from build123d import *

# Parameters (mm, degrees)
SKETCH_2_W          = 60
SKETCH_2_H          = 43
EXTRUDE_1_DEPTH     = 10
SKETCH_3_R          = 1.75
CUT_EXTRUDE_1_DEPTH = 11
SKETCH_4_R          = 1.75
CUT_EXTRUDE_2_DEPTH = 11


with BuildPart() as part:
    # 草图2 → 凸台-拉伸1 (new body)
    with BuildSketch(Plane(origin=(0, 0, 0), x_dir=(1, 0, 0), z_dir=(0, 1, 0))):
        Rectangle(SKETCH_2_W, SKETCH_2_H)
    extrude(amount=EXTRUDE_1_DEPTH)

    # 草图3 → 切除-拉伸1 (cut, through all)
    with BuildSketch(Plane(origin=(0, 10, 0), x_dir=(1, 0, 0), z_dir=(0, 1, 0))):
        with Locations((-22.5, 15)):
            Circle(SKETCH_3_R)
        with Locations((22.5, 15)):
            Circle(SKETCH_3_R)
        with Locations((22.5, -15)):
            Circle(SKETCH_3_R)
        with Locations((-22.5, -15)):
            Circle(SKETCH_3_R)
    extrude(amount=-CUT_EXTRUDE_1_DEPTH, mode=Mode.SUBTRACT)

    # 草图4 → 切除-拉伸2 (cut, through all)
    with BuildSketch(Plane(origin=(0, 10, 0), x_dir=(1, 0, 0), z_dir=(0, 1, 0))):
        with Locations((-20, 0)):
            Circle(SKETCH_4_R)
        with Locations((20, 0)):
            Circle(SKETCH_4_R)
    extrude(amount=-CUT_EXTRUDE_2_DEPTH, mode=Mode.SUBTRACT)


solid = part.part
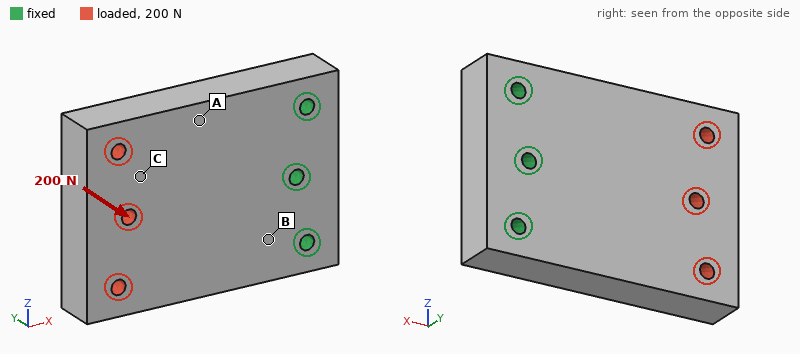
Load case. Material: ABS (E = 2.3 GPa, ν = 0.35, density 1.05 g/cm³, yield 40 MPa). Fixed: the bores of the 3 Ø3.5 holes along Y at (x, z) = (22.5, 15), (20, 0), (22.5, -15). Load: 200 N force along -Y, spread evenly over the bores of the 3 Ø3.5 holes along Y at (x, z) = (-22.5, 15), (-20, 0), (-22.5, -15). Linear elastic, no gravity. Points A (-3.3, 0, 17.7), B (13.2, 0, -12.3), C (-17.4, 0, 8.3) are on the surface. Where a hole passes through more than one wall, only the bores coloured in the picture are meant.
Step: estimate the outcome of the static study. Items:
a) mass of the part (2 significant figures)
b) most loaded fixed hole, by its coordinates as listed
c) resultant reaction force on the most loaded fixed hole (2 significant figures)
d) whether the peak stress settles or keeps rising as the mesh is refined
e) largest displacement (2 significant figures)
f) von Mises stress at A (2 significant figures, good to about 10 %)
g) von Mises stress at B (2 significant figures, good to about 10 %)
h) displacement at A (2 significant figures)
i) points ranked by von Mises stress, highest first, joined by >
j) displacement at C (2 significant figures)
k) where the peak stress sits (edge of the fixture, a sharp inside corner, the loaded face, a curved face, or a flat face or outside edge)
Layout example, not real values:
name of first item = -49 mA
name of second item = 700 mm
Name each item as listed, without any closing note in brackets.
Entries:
mass of the part = 26 g
most loaded fixed hole, by its coordinates as listed = (20, 0)
resultant reaction force on the most loaded fixed hole = 210 N
whether the peak stress settles or keeps rising as the mesh is refined = keeps rising
largest displacement = 0.87 mm
von Mises stress at A = 5.1 MPa
von Mises stress at B = 8.8 MPa
displacement at A = 0.29 mm
points ranked by von Mises stress, highest first, joined by > = B > A > C
displacement at C = 0.59 mm
where the peak stress sits = edge of the fixture
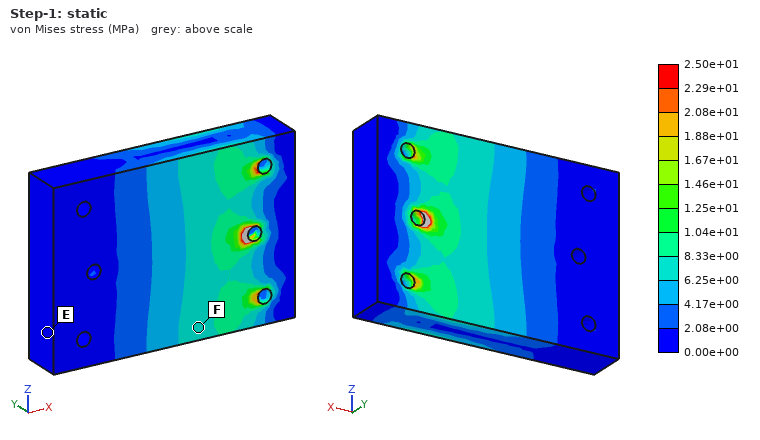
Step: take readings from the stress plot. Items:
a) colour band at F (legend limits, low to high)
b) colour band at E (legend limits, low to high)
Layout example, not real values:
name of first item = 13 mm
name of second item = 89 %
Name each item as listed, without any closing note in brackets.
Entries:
colour band at F = 6.25e+00 to 8.33e+00 MPa
colour band at E = 0.00e+00 to 2.08e+00 MPa
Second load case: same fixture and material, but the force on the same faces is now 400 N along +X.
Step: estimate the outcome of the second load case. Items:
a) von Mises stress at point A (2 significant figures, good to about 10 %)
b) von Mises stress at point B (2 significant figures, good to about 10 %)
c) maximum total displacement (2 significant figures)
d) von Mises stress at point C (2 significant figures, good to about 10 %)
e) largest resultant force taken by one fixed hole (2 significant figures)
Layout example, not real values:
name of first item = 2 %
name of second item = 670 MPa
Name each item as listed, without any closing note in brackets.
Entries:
von Mises stress at point A = 0.88 MPa
von Mises stress at point B = 0.94 MPa
maximum total displacement = 21 µm
von Mises stress at point C = 0.68 MPa
largest resultant force taken by one fixed hole = 140 N
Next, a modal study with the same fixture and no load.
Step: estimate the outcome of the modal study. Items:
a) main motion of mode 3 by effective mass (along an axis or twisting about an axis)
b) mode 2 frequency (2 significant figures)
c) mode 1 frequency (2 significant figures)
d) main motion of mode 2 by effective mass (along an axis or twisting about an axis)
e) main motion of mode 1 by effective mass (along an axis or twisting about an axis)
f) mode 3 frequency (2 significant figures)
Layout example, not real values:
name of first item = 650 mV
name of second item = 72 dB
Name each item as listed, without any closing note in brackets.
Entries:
main motion of mode 3 by effective mass = along Z
mode 2 frequency = 2200 Hz
mode 1 frequency = 890 Hz
main motion of mode 2 by effective mass = twisting about X
main motion of mode 1 by effective mass = along Y
mode 3 frequency = 2600 Hz
